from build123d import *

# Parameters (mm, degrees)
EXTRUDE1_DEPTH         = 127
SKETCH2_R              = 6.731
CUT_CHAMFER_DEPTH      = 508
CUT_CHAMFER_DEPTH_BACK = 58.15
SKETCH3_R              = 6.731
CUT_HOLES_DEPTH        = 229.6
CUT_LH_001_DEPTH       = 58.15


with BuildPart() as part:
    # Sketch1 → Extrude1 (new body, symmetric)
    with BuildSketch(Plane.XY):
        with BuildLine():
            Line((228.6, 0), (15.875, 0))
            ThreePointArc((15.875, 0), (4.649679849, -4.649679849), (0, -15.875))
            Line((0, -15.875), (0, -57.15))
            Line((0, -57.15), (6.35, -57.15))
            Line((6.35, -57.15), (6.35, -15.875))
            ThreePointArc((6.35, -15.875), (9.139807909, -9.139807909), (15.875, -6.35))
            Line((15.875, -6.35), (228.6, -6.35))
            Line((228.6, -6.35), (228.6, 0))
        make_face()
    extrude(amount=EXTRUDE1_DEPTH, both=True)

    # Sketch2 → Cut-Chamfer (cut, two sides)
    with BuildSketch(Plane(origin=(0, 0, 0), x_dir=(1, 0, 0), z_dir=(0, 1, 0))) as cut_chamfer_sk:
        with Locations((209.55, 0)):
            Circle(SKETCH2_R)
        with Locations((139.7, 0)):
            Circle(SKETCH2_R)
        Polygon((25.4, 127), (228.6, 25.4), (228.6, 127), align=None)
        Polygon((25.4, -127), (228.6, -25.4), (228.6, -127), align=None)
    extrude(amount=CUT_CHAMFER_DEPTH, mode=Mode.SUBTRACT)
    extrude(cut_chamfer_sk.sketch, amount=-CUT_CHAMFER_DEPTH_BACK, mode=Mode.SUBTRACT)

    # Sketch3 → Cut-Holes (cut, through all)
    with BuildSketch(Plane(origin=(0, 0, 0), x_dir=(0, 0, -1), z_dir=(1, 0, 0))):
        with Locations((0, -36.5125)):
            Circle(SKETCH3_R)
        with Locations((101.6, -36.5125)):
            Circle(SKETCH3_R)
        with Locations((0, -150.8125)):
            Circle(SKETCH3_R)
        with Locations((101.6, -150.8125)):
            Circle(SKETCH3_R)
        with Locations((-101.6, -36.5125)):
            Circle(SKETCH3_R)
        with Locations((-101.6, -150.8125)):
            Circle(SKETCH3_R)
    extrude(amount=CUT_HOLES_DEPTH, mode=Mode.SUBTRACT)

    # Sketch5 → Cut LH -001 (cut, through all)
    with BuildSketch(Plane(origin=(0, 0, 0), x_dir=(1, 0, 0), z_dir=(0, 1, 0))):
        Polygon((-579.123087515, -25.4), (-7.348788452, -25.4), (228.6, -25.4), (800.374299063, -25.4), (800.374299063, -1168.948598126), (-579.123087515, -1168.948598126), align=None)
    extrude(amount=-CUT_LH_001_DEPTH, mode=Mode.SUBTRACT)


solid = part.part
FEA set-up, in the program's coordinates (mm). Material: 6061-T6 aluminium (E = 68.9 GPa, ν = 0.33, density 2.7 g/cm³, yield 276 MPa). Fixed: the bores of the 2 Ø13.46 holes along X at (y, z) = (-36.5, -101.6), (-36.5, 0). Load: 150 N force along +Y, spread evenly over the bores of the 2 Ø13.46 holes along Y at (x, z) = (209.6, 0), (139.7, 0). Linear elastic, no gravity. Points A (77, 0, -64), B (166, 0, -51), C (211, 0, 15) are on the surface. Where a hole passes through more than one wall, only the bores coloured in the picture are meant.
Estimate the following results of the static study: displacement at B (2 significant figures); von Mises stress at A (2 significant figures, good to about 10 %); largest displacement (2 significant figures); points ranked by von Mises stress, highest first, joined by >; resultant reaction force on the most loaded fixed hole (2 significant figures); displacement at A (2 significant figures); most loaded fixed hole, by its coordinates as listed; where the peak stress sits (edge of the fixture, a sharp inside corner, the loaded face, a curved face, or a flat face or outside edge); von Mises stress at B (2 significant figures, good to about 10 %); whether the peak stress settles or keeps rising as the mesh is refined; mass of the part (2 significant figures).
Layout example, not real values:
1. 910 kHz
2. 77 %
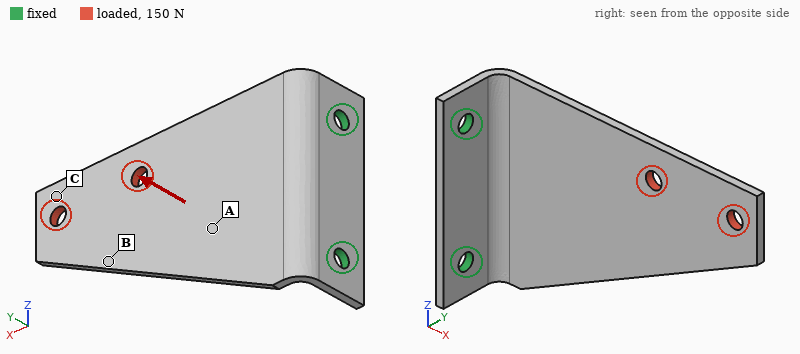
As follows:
1. 1.6 mm
2. 18 MPa
3. 2.9 mm
4. A > B > C
5. 150 N
6. 0.47 mm
7. (-36.5, 0)
8. edge of the fixture
9. 8.9 MPa
10. keeps rising
11. 530 g
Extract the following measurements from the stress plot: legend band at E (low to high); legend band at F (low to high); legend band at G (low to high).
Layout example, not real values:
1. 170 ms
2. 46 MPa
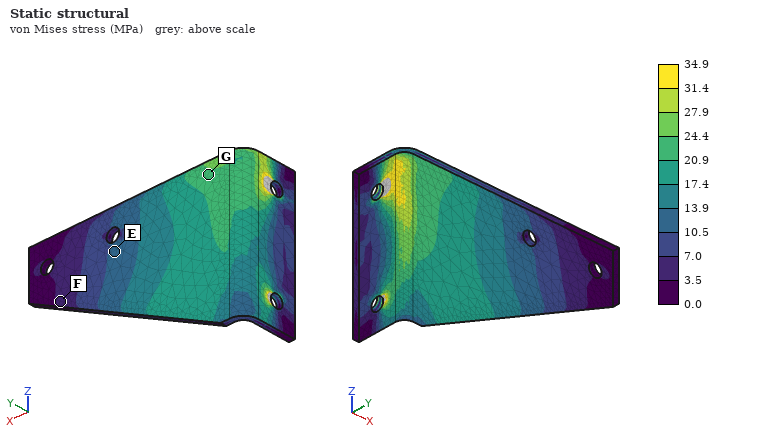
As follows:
1. 10.5 to 13.9 MPa
2. 3.5 to 7.0 MPa
3. 20.9 to 24.4 MPa
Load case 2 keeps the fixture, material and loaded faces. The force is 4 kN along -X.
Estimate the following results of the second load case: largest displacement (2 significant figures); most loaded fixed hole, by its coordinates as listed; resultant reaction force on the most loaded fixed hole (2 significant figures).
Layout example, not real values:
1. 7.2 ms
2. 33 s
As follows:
1. 2.7 mm
2. (-36.5, 0)
3. 3.9 kN
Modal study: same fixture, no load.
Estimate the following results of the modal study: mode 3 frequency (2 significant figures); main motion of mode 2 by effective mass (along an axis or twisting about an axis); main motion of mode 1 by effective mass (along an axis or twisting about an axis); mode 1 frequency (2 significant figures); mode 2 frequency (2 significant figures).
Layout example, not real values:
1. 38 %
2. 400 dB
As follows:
1. 570 Hz
2. along Z
3. along Y
4. 120 Hz
5. 520 Hz
